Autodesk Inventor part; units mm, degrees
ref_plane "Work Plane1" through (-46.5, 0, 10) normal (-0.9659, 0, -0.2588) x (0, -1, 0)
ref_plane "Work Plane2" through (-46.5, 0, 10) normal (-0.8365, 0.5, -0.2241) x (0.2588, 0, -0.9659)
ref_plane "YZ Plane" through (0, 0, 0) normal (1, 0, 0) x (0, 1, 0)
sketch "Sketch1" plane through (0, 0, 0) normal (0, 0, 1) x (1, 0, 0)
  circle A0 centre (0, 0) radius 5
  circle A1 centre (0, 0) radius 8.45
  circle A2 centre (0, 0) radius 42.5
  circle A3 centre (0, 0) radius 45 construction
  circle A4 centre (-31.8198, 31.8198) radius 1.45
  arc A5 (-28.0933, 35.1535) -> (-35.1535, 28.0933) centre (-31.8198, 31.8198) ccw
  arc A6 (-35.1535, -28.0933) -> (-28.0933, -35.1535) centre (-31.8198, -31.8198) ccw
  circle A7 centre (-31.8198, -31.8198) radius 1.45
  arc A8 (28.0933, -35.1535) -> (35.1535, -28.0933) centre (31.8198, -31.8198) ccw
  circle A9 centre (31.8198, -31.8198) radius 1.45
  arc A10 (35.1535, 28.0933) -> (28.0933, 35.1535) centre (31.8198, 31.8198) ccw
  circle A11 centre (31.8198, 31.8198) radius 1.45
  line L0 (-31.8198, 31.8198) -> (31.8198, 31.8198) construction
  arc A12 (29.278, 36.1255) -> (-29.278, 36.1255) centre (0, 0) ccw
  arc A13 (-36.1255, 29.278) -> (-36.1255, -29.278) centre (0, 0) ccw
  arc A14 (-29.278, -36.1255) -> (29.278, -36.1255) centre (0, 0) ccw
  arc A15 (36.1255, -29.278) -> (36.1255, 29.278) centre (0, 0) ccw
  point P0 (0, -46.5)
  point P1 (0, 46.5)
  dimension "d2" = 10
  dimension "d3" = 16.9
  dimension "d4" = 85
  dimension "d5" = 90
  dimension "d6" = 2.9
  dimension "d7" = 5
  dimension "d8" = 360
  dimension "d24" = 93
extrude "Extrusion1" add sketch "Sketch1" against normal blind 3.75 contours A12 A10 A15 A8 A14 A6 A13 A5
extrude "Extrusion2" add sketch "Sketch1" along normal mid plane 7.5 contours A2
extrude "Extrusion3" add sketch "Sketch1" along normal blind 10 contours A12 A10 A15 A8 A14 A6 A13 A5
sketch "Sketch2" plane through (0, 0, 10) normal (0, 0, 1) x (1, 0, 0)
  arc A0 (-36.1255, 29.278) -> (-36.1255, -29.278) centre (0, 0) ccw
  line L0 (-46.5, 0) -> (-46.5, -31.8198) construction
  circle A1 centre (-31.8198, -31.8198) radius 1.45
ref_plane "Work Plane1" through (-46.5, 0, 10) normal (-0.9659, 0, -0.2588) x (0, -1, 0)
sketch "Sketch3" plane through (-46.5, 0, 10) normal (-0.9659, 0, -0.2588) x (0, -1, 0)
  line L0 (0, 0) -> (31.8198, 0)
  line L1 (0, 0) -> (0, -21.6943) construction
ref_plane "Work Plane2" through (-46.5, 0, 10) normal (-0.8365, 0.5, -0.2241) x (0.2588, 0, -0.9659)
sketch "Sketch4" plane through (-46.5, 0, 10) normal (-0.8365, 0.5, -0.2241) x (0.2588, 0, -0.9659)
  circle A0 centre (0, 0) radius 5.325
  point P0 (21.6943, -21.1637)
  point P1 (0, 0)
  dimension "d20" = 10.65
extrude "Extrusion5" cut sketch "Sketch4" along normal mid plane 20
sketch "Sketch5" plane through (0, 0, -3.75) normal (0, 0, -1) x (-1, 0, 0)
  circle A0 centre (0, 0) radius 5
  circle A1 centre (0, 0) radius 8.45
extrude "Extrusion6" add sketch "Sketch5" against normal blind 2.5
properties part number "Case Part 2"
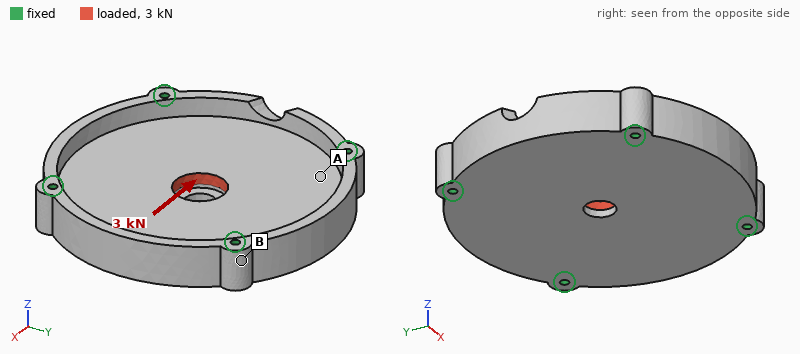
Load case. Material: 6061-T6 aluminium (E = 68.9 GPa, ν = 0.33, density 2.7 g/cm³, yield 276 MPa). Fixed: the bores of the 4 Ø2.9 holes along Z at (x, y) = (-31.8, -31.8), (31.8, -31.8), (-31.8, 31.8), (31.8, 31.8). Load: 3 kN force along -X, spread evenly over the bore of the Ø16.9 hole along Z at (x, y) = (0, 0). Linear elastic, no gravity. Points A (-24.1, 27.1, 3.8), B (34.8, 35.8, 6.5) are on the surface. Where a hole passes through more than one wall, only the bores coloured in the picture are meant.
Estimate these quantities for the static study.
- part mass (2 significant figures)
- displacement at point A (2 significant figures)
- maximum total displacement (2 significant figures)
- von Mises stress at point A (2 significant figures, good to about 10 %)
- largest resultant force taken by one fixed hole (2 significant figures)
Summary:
160 g
1.1 µm
5.5 µm
7.3 MPa
780 N
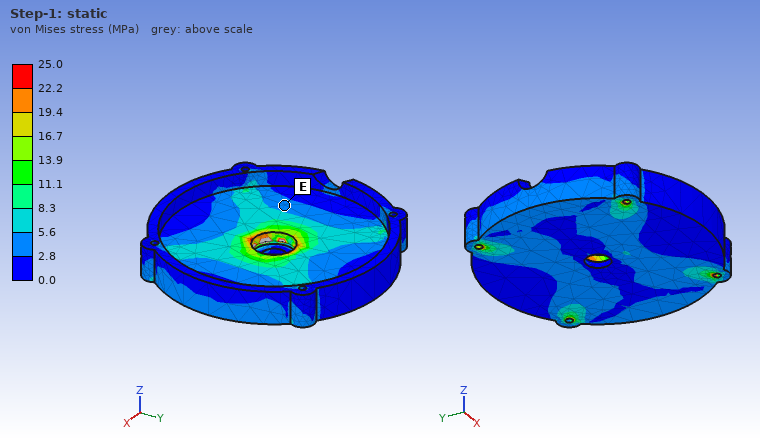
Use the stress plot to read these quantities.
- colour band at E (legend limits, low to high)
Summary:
2.8 to 5.6 MPa
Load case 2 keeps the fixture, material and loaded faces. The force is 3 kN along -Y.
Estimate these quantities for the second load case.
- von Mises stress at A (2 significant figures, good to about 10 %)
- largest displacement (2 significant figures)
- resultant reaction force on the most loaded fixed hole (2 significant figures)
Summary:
6.4 MPa
5.5 µm
770 N
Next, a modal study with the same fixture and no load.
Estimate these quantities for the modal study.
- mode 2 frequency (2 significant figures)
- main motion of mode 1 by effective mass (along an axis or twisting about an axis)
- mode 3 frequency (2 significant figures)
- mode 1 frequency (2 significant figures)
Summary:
9700 Hz
along Z
9800 Hz
6200 Hz
